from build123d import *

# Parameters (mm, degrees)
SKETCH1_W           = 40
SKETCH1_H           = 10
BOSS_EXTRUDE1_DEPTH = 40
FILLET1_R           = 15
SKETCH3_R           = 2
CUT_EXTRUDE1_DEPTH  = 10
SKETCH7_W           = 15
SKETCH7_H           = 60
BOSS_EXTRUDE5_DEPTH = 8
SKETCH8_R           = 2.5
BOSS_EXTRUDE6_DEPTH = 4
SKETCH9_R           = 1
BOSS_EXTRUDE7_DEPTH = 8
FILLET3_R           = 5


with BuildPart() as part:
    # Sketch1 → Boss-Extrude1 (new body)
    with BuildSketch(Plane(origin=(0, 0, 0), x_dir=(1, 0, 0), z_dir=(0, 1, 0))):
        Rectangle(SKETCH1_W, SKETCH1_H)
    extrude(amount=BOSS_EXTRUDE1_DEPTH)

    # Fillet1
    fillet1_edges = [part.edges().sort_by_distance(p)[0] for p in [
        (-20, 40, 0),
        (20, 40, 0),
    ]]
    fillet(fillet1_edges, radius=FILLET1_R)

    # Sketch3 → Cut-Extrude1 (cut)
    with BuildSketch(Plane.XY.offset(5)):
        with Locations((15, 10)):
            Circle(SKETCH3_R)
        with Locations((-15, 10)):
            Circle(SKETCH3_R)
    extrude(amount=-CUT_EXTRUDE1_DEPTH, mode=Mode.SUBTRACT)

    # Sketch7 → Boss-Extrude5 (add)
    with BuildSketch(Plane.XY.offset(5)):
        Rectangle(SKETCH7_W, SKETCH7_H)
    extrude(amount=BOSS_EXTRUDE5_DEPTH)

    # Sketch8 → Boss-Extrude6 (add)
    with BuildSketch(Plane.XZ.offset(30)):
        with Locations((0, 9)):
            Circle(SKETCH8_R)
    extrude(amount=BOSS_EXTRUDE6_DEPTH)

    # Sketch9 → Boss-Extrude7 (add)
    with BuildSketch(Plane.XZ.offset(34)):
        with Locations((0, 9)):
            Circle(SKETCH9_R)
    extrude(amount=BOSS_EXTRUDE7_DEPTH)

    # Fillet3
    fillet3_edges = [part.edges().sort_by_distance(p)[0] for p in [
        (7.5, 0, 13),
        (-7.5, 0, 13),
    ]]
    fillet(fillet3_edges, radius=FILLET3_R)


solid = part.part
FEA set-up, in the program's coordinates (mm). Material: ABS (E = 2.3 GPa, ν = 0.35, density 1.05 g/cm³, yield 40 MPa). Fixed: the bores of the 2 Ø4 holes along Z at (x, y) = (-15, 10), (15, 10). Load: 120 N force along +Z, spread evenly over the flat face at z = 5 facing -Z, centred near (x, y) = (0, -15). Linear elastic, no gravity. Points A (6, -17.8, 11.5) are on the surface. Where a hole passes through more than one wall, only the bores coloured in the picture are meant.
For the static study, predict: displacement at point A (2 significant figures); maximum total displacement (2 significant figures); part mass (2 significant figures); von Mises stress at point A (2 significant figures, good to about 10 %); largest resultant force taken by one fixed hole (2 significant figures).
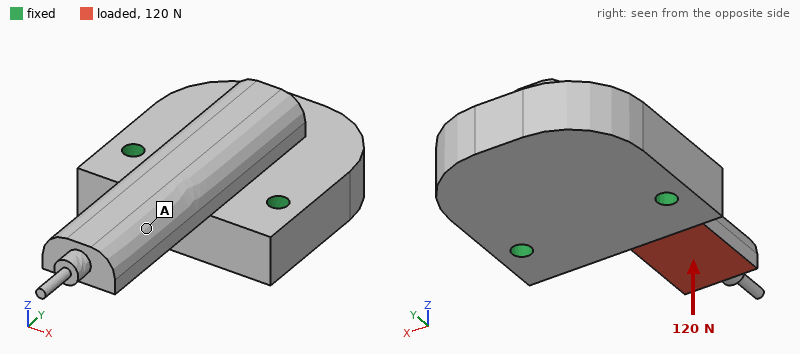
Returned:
0.41 mm
0.98 mm
23 g
1.8 MPa
75 N
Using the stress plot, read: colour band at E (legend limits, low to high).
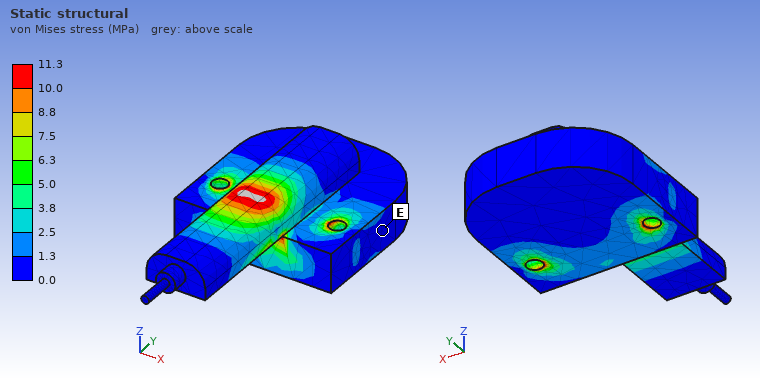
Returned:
0.0 to 1.3 MPa
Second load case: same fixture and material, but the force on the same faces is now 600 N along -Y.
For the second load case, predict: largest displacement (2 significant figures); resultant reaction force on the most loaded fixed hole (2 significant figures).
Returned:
0.88 mm
300 N
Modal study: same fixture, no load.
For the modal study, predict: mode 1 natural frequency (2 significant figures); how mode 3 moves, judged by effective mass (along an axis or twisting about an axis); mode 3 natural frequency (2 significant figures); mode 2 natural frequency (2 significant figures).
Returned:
1300 Hz
along Z
2500 Hz
2100 Hz
